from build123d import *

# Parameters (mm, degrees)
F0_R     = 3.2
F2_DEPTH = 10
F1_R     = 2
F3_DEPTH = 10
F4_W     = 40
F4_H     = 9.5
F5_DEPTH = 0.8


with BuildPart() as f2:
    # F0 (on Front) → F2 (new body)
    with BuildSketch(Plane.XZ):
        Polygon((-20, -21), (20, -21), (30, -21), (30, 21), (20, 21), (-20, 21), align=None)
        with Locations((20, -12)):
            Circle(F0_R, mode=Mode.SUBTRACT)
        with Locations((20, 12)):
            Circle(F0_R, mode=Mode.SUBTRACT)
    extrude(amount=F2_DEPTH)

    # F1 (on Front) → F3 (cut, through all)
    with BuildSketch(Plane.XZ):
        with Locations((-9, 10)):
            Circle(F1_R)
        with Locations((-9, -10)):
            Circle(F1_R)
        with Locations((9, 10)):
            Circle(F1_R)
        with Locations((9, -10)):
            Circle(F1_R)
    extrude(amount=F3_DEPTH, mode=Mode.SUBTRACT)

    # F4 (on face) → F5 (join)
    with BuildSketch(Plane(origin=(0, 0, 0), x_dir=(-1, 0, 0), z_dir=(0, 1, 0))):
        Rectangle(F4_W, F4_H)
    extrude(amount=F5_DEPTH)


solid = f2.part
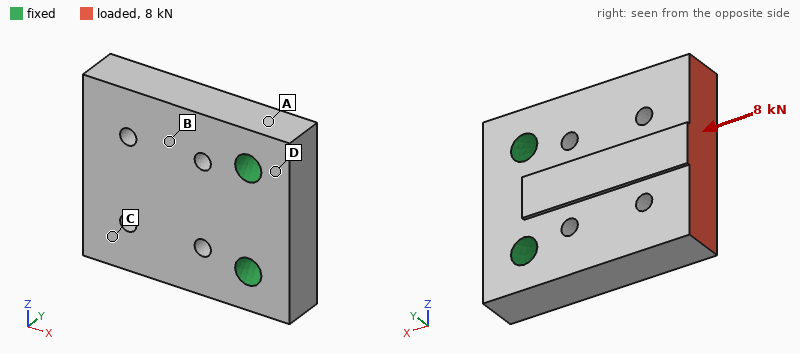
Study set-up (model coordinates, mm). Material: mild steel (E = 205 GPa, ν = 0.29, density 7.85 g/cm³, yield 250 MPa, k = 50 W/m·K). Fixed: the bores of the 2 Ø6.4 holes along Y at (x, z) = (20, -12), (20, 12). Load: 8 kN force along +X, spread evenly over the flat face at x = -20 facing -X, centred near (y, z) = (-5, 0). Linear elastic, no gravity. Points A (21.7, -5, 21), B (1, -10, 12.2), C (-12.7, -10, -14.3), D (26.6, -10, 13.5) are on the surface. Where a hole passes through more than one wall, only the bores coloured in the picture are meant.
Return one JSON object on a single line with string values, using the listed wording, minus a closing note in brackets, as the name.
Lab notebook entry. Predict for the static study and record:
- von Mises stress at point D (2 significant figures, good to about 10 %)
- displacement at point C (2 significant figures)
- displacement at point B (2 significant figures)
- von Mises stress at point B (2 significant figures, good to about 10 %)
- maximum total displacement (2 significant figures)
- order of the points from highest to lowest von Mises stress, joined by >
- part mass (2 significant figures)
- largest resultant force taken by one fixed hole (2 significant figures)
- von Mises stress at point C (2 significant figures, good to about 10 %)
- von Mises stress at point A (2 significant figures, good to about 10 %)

{"von Mises stress at point D": "5.2 MPa", "displacement at point C": "3.5 µm", "displacement at point B": "2.1 µm", "von Mises stress at point B": "17 MPa", "maximum total displacement": "4.3 µm", "order of the points from highest to lowest von Mises stress, joined by >": "C > B > A > D", "part mass": "160 g", "largest resultant force taken by one fixed hole": "4.0 kN", "von Mises stress at point C": "24 MPa", "von Mises stress at point A": "10 MPa"}
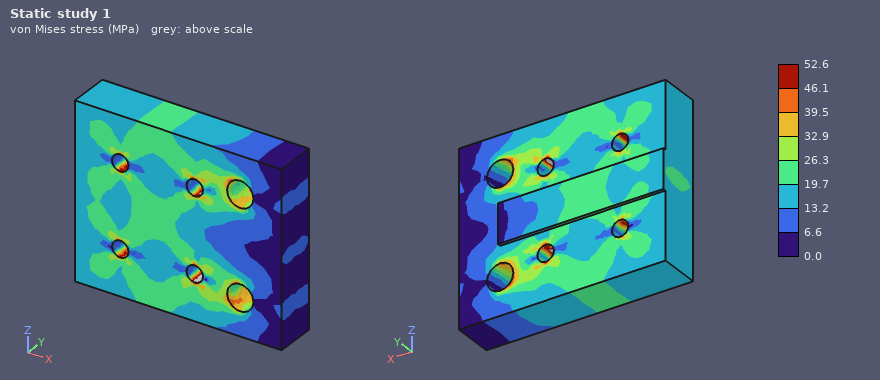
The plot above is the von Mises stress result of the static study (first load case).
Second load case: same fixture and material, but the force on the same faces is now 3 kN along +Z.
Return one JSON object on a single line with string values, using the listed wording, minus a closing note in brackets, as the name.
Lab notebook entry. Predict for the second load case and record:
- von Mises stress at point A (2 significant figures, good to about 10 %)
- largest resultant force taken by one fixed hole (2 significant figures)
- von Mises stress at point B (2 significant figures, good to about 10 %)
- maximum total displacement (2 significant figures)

{"von Mises stress at point A": "18 MPa", "largest resultant force taken by one fixed hole": "4.4 kN", "von Mises stress at point B": "20 MPa", "maximum total displacement": "12 µm"}
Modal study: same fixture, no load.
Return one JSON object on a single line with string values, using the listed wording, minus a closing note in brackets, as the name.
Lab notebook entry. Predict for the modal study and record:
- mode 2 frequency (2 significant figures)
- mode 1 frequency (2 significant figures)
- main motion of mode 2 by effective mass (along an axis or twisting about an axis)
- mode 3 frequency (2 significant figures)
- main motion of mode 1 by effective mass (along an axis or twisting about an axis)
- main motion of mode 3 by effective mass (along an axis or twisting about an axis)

{"mode 2 frequency": "11 kHz", "mode 1 frequency": "5000 Hz", "main motion of mode 2 by effective mass": "twisting about X", "mode 3 frequency": "13 kHz", "main motion of mode 1 by effective mass": "along Y", "main motion of mode 3 by effective mass": "along Z"}
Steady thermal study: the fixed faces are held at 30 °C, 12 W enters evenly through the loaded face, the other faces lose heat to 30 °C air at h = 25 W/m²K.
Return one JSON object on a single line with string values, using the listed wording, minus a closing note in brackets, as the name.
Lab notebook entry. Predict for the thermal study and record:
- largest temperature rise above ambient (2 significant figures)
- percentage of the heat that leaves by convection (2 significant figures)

{"largest temperature rise above ambient": "22 K", "percentage of the heat that leaves by convection": "11 %"}
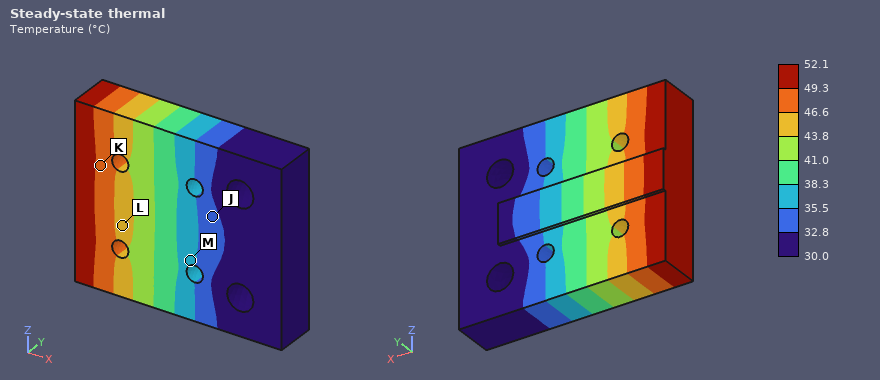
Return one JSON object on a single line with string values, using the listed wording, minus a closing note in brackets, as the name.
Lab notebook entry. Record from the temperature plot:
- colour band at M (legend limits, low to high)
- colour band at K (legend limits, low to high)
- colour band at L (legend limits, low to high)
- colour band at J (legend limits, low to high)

{"colour band at M": "35.5 to 38.3 °C", "colour band at K": "46.6 to 49.3 °C", "colour band at L": "43.8 to 46.6 °C", "colour band at J": "32.8 to 35.5 °C"}
